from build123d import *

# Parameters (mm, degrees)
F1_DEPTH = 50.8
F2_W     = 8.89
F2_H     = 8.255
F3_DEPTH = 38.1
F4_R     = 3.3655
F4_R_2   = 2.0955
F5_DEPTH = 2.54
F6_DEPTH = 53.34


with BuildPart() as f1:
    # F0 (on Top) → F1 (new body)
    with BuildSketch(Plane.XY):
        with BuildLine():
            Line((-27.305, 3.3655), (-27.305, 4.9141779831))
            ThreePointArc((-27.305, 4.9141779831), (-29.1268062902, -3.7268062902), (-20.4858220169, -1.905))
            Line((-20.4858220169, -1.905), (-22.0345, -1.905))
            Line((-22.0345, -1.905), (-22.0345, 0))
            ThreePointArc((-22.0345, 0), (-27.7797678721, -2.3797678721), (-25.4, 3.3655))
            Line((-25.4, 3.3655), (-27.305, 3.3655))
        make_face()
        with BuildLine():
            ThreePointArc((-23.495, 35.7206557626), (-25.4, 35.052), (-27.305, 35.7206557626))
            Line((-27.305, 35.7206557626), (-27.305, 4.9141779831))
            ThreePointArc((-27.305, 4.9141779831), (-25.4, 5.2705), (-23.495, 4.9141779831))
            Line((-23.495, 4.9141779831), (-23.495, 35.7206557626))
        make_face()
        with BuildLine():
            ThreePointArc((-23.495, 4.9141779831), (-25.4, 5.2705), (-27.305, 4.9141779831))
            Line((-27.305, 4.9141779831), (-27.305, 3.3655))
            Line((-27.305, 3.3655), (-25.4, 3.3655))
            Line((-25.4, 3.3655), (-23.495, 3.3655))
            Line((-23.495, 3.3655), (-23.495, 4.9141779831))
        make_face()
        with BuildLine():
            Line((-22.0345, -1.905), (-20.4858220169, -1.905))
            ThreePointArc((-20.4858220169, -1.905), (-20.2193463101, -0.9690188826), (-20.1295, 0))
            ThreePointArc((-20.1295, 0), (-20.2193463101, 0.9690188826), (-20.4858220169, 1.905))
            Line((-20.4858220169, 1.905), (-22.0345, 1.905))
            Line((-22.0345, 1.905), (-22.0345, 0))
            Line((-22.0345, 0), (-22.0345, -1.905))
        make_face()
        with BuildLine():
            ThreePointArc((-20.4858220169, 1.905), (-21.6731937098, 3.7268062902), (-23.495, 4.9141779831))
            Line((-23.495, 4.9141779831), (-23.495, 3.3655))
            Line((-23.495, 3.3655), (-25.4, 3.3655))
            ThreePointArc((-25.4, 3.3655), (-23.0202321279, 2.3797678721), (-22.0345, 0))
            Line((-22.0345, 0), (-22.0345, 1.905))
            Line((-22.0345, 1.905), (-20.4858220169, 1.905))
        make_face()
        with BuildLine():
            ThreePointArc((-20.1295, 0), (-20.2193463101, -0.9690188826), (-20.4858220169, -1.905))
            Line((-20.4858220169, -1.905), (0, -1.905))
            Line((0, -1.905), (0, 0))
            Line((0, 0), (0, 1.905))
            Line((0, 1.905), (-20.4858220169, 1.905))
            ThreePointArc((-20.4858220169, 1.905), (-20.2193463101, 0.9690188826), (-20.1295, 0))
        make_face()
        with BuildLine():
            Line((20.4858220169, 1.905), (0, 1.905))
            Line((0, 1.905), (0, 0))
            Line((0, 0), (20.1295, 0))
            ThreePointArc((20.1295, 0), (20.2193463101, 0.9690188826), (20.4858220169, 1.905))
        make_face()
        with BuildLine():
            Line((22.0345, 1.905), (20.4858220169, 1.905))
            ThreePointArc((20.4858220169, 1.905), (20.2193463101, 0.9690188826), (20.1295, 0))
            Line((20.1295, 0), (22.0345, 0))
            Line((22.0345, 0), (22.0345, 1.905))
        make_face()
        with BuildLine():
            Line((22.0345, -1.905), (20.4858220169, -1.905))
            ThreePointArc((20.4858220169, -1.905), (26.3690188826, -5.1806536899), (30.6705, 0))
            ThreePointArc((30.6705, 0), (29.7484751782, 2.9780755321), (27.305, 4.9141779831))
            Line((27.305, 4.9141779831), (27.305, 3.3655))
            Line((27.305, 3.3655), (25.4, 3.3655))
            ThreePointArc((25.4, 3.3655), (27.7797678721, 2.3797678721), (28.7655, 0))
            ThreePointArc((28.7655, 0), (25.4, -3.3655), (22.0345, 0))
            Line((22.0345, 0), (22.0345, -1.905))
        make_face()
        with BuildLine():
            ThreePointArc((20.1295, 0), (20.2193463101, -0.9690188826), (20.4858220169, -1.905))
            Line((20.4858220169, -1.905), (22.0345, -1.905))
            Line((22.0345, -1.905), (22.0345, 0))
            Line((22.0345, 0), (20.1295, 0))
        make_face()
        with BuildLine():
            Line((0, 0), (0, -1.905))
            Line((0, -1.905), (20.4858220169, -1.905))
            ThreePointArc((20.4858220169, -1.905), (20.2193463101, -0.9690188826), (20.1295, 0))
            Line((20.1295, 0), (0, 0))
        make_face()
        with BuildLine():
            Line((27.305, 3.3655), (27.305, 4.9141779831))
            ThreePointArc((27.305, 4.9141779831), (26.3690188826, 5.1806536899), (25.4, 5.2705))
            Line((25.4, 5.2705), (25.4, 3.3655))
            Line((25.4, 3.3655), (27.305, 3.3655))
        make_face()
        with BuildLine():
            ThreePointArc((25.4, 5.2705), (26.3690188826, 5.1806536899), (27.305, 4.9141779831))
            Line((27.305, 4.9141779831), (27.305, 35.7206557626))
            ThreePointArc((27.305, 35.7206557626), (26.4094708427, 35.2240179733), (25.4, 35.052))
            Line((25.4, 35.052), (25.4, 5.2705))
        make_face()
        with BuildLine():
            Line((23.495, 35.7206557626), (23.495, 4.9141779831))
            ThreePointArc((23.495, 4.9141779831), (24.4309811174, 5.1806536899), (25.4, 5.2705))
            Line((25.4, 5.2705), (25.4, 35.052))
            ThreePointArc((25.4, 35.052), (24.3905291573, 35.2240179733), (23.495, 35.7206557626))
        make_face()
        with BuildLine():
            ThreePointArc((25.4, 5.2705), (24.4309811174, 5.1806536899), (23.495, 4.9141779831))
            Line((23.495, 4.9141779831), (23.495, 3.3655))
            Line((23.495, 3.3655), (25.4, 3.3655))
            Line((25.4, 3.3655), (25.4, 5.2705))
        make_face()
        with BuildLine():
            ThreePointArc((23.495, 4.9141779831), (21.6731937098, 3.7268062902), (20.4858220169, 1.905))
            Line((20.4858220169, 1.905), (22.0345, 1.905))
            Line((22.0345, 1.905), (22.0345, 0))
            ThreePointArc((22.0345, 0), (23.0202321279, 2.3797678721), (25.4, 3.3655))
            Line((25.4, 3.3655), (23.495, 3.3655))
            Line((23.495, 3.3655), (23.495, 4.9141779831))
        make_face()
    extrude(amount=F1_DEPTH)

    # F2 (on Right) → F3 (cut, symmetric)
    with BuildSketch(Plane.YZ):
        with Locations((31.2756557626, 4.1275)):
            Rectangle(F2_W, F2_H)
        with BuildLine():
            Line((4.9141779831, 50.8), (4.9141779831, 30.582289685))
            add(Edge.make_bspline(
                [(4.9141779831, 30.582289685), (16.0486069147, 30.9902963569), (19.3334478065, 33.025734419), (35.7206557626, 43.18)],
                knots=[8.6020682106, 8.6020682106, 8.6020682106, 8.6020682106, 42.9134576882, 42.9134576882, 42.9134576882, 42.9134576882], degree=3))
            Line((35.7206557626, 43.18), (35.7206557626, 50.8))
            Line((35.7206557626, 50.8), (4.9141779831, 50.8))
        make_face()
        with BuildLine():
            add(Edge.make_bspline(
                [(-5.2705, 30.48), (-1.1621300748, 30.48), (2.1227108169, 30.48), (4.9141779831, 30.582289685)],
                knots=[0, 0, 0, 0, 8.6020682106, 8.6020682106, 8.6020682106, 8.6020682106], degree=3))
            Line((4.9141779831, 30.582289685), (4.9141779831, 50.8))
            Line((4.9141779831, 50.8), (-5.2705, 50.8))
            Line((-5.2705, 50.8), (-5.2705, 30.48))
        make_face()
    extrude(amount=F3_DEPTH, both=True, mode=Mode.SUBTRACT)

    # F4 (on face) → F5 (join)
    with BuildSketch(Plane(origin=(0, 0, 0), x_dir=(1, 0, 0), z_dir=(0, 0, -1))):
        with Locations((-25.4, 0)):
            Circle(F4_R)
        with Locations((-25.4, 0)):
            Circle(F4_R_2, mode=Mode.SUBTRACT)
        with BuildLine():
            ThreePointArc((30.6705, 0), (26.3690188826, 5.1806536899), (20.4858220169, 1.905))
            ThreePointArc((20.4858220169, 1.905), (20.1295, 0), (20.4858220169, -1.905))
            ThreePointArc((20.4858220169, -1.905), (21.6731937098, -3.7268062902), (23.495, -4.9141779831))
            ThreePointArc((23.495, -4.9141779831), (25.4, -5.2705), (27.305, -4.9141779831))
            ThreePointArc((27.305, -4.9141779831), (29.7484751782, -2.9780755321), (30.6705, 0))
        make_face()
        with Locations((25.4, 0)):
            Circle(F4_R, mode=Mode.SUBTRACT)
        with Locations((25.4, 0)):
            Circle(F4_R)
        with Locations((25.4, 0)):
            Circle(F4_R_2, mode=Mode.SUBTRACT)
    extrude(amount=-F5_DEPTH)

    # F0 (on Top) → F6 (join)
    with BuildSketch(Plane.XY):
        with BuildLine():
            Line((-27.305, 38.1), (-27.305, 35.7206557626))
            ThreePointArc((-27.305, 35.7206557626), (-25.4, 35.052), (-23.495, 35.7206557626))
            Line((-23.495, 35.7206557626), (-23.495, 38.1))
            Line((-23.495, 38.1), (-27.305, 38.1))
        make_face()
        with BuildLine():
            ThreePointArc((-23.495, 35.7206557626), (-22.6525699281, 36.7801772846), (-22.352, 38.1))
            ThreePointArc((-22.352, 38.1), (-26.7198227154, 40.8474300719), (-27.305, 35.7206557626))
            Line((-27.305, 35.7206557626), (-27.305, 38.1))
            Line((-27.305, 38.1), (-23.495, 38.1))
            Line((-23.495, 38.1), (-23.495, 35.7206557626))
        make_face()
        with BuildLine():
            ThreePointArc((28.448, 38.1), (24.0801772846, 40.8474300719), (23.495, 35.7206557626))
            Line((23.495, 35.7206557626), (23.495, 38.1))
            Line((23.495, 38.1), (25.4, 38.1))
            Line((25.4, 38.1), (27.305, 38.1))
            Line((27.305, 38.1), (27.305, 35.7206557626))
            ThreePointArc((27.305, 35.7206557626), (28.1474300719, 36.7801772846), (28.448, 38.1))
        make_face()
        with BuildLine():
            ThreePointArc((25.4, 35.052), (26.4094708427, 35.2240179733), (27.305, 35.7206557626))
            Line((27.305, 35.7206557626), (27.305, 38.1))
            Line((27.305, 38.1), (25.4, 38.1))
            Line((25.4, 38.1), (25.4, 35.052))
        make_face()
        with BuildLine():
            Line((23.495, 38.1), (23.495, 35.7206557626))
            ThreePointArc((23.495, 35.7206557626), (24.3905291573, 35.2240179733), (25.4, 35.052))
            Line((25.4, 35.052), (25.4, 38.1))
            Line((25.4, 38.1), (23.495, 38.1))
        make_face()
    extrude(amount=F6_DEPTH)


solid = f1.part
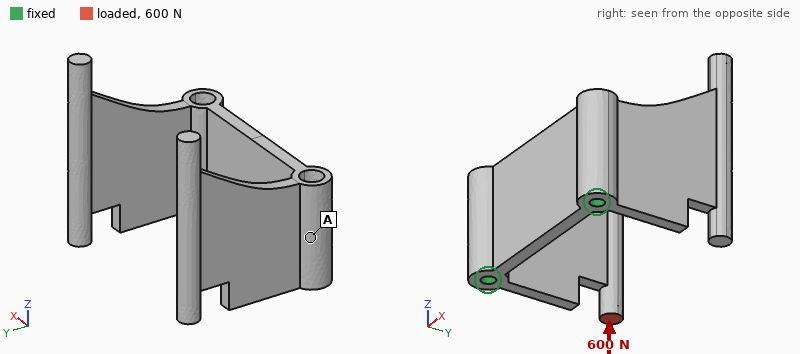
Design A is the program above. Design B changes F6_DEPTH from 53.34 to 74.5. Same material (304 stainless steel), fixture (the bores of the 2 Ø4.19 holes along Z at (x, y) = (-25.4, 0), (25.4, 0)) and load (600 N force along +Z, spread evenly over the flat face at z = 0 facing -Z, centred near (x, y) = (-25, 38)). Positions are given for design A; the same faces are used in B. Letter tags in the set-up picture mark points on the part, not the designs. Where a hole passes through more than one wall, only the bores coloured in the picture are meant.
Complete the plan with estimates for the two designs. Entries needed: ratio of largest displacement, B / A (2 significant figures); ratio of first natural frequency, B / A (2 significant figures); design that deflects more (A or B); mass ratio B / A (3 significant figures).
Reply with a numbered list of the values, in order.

1. 1.3
2. 0.76
3. B
4. 1.07
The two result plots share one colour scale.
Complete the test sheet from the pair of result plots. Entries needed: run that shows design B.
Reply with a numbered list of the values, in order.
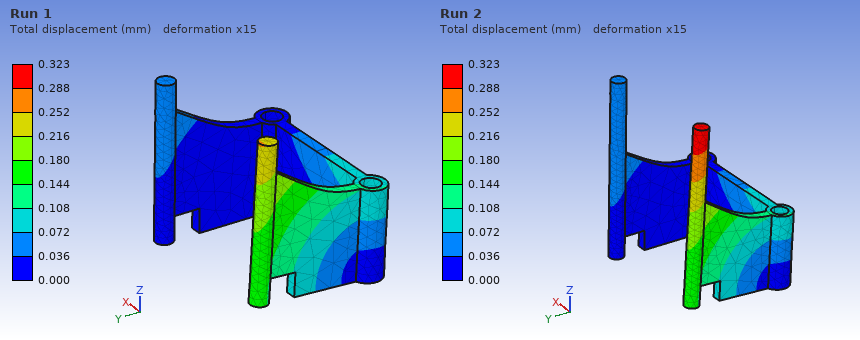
1. Run 2
